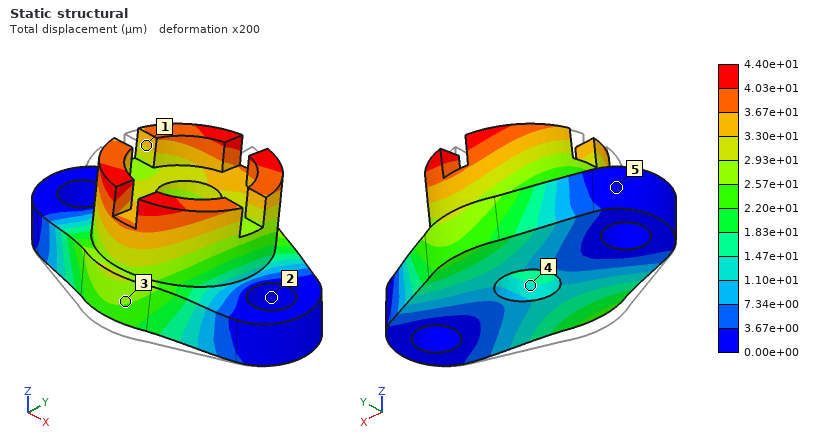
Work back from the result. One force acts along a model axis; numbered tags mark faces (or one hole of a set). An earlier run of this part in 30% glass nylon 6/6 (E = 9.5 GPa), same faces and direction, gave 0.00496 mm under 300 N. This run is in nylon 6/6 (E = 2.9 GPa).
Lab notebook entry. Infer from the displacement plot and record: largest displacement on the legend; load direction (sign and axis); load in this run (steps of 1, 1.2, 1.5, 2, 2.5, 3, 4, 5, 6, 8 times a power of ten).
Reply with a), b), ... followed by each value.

a) 4.40e+01 µm
b) +Y
c) 800 N
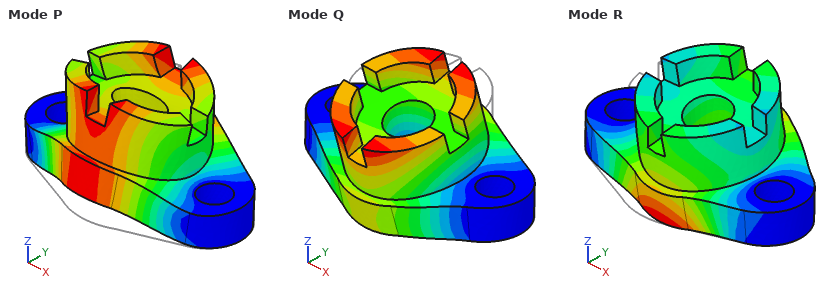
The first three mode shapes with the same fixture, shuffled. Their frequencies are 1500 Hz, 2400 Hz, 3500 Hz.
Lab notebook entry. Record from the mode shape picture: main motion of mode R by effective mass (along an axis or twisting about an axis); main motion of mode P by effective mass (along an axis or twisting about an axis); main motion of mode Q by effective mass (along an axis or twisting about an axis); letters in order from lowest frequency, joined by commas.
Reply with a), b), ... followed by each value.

a) along Y
b) along Z
c) along Y
d) Q, P, R
